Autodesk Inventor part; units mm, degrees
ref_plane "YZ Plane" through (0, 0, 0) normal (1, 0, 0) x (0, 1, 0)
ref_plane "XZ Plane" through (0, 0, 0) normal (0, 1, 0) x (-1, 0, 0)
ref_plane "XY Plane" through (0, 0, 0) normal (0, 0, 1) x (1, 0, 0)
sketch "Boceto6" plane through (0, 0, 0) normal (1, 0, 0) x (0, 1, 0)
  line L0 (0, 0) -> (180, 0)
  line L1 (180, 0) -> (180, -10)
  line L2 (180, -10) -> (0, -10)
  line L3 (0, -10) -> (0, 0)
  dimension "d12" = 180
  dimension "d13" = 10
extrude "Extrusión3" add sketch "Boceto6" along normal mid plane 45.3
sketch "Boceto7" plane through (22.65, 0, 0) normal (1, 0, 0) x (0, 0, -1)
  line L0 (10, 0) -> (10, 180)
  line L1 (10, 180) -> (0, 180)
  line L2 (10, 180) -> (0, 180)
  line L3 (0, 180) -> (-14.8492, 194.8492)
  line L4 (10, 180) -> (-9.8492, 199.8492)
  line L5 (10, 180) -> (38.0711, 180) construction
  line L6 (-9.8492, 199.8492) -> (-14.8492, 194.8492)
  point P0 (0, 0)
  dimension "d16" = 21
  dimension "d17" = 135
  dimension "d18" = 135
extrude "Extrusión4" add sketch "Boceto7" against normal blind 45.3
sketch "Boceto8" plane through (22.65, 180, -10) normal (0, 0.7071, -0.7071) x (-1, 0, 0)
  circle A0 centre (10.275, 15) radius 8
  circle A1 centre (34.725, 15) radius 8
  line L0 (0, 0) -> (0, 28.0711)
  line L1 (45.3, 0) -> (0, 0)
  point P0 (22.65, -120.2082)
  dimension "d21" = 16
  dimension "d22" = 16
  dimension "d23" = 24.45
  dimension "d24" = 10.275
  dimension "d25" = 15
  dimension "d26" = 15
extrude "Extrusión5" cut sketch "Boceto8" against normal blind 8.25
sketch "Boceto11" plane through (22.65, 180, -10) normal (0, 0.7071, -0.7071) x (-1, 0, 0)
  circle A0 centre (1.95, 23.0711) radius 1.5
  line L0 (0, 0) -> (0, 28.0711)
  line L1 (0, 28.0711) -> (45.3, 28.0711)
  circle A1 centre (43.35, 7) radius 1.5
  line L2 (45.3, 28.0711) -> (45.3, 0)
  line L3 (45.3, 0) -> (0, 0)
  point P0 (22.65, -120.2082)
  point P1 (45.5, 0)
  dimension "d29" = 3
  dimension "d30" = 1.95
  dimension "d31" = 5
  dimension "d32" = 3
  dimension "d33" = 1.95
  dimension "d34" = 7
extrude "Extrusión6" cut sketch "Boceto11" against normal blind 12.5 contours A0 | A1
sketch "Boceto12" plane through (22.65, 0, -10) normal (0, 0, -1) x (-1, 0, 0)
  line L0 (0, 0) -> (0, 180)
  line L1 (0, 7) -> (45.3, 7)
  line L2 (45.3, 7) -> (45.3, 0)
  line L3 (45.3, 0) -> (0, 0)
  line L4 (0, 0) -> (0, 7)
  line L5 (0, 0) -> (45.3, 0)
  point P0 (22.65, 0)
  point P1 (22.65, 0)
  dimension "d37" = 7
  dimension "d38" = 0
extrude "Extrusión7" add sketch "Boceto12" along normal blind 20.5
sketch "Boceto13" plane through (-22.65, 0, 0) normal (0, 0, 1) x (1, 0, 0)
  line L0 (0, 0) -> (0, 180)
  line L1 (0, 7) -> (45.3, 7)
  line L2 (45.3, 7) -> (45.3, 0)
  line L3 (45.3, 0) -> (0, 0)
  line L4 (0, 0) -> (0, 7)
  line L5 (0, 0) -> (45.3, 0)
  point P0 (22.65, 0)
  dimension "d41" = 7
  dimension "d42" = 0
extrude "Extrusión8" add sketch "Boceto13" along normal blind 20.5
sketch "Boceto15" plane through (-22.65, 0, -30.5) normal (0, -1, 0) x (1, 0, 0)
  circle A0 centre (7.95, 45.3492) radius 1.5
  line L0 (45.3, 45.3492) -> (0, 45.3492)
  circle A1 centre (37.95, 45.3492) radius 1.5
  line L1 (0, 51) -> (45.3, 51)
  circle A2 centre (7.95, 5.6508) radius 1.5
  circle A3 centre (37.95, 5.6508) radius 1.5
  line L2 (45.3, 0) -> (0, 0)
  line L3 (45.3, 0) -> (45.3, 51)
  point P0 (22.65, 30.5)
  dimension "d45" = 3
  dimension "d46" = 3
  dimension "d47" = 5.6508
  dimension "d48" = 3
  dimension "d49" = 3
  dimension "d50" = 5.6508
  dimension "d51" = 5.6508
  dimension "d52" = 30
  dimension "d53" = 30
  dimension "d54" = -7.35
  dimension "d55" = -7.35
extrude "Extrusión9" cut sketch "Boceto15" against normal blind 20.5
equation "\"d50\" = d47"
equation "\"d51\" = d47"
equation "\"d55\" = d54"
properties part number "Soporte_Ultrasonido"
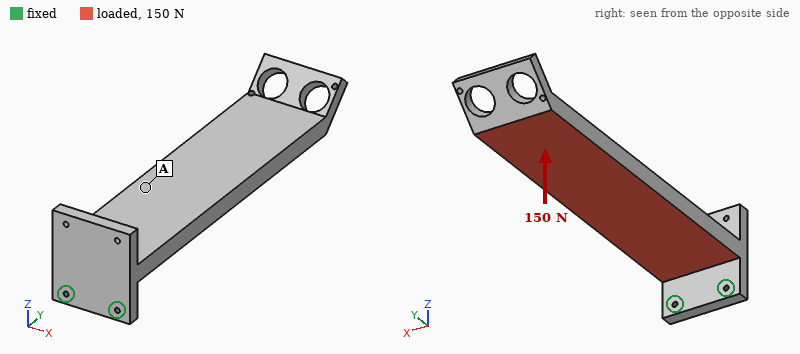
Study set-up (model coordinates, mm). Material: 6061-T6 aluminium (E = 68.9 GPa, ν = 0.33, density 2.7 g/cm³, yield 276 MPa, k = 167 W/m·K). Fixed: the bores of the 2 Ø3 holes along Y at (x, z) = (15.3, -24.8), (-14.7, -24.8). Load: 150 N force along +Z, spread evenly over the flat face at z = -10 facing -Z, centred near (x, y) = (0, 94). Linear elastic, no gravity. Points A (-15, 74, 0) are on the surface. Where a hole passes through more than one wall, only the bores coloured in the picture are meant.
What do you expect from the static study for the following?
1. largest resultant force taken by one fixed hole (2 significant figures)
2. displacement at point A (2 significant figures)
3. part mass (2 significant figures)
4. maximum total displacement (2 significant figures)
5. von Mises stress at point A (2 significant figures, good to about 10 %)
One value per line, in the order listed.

87 N
0.31 mm
270 g
1.1 mm
6.4 MPa
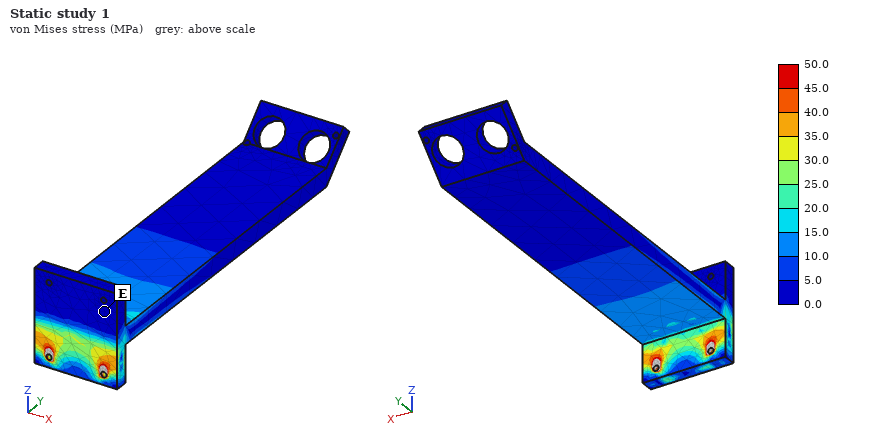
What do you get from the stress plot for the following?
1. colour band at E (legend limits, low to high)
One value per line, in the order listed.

0.0 to 5.0 MPa
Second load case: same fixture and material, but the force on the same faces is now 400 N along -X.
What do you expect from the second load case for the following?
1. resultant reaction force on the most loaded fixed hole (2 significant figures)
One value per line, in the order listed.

1.1 kN
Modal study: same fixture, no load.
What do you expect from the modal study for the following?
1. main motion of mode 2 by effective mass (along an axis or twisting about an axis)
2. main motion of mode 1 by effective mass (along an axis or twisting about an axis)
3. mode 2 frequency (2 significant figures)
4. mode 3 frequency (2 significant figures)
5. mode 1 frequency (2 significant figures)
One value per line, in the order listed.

along X
along Z
410 Hz
1100 Hz
150 Hz
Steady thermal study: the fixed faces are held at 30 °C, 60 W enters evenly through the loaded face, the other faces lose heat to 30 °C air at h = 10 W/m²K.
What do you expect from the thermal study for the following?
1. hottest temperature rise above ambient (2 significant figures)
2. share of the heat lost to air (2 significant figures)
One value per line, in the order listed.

77 K
16 %
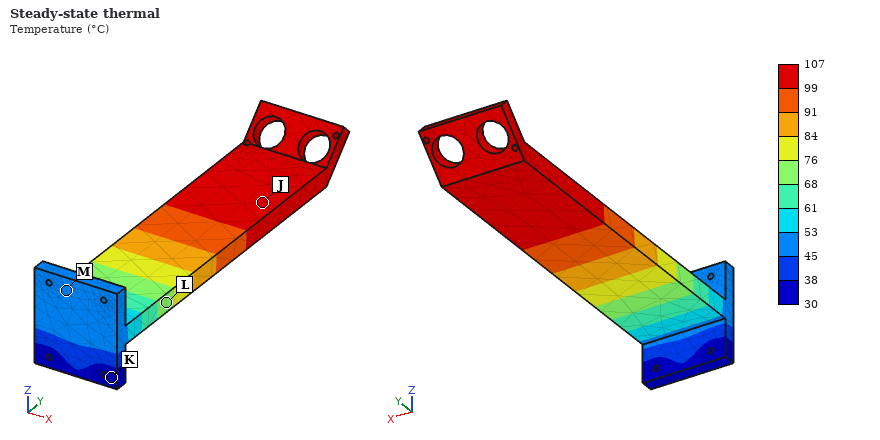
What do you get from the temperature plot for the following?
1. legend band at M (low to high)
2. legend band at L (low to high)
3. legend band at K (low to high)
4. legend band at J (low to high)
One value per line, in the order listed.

45 to 53 °C
68 to 76 °C
30 to 38 °C
99 to 107 °C
